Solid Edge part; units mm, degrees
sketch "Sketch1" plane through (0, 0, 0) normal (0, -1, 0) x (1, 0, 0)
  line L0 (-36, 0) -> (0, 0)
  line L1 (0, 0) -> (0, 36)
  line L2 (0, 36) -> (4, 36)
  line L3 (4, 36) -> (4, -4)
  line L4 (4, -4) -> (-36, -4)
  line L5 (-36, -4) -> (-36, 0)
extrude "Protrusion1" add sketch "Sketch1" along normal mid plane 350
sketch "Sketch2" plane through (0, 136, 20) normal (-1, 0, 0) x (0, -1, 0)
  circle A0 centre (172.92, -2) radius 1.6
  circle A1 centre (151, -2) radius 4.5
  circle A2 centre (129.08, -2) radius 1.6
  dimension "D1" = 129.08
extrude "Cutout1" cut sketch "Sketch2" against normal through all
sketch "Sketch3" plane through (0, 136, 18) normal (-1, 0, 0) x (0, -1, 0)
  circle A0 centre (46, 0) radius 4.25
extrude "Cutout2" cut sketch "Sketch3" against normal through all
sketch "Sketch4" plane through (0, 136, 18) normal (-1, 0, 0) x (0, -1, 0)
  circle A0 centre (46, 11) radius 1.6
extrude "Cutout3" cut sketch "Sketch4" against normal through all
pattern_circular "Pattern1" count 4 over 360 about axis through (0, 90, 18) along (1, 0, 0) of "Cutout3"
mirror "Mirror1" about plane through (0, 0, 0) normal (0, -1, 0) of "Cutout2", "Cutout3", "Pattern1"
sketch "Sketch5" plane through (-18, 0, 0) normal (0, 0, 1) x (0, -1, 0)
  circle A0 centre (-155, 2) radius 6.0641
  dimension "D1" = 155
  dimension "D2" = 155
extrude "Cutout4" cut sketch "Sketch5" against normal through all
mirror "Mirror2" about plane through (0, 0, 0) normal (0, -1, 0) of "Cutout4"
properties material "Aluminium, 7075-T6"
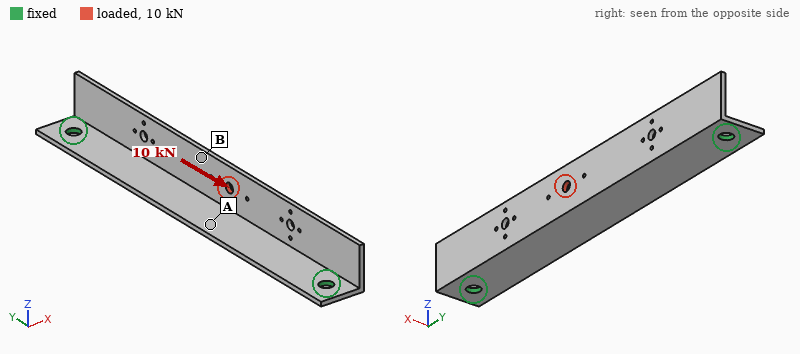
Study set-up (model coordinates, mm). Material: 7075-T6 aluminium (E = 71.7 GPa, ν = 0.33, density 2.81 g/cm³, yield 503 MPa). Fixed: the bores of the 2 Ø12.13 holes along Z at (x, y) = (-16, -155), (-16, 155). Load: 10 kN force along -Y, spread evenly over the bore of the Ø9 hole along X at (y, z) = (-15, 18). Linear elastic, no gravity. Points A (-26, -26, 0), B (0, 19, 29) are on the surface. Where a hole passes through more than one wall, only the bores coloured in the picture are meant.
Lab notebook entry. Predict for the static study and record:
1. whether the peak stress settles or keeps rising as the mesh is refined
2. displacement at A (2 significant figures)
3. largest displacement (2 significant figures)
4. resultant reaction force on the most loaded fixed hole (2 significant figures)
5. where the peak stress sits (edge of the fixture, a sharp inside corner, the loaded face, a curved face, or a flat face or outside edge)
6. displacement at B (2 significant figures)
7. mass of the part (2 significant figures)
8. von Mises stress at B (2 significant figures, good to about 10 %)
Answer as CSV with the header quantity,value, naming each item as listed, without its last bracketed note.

quantity,value
whether the peak stress settles or keeps rising as the mesh is refined,keeps rising
displacement at A,0.039 mm
largest displacement,0.14 mm
resultant reaction force on the most loaded fixed hole,5.2 kN
where the peak stress sits,a sharp inside corner
displacement at B,0.060 mm
mass of the part,290 g
von Mises stress at B,34 MPa
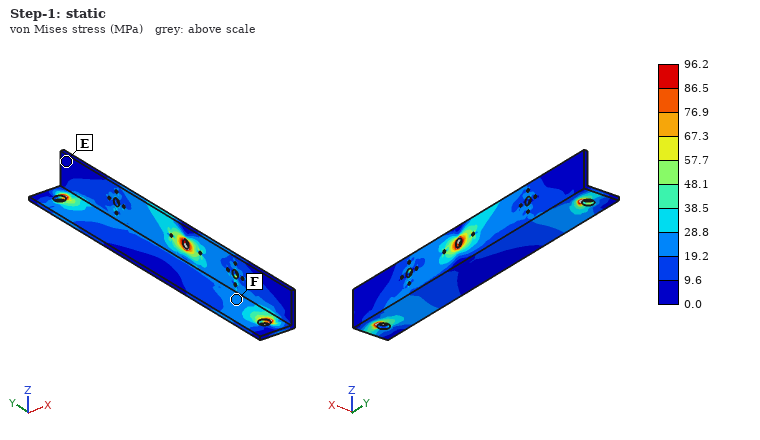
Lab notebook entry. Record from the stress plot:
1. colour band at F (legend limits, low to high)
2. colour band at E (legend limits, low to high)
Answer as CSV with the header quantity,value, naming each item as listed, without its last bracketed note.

quantity,value
colour band at F,19.2 to 28.8 MPa
colour band at E,0.0 to 9.6 MPa
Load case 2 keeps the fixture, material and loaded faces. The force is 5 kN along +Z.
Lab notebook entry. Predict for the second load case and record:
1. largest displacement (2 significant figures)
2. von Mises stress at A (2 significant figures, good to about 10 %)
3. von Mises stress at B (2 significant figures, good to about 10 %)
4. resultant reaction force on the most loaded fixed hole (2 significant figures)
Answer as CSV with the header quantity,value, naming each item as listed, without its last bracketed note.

quantity,value
largest displacement,1.5 mm
von Mises stress at A,33 MPa
von Mises stress at B,150 MPa
resultant reaction force on the most loaded fixed hole,6.4 kN
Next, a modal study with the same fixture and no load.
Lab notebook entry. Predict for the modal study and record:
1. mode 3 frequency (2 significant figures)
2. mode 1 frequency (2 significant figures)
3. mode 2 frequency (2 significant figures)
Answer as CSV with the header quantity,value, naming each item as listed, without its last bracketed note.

quantity,value
mode 3 frequency,1100 Hz
mode 1 frequency,540 Hz
mode 2 frequency,860 Hz
